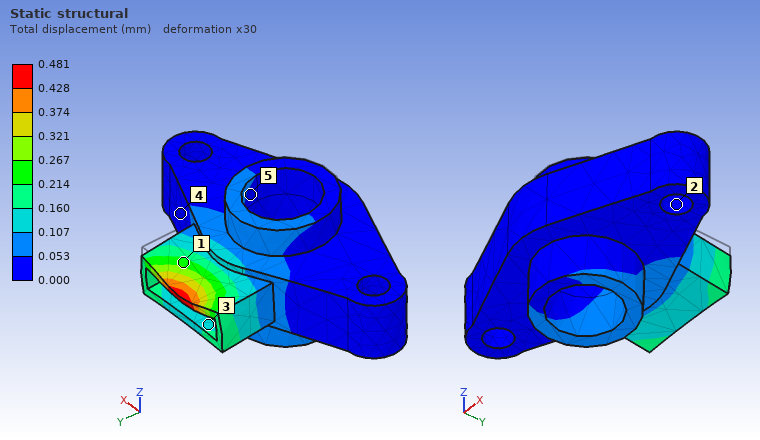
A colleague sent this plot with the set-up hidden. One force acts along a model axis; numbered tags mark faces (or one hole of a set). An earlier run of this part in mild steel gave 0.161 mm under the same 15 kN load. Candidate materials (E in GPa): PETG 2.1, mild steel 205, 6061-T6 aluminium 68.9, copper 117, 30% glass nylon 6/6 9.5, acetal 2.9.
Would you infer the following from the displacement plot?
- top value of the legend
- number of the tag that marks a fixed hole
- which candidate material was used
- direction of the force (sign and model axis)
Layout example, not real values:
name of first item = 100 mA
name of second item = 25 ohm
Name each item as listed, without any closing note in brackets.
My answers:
top value of the legend = 0.481 mm
number of the tag that marks a fixed hole = 2
which candidate material was used = 6061-T6 aluminium
direction of the force = -Z
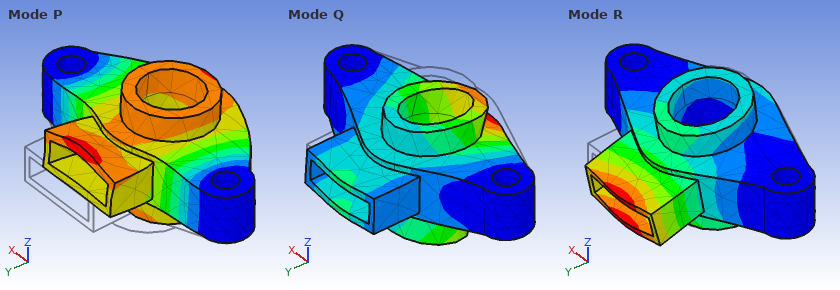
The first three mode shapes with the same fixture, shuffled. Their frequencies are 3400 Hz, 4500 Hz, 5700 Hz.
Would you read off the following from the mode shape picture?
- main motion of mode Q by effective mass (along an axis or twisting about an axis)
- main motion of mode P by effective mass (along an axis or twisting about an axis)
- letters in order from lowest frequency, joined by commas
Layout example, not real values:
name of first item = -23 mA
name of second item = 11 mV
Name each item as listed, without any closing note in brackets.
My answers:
main motion of mode Q by effective mass = along Z
main motion of mode P by effective mass = along Y
letters in order from lowest frequency, joined by commas = R, Q, P
